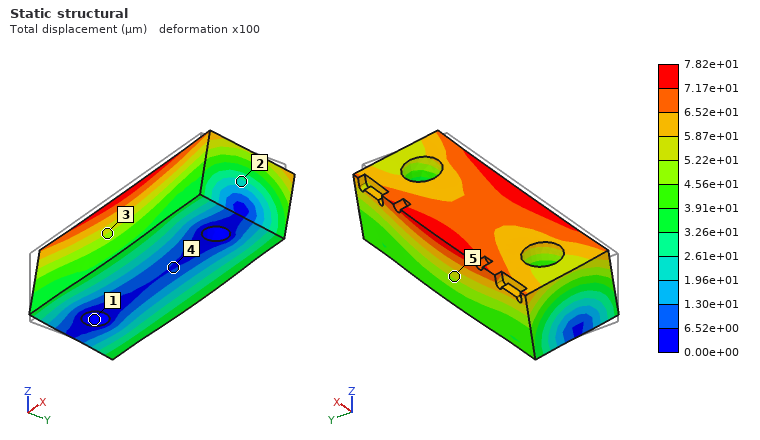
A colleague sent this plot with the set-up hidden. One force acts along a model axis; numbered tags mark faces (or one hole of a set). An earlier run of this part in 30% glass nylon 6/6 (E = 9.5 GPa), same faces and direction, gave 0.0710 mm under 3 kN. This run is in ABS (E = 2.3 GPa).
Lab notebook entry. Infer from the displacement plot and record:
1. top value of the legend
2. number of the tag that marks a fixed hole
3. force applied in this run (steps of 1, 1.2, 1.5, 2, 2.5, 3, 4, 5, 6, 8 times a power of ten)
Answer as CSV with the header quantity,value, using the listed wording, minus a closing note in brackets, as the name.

quantity,value
top value of the legend,7.82e+01 µm
number of the tag that marks a fixed hole,1
force applied in this run,800 N
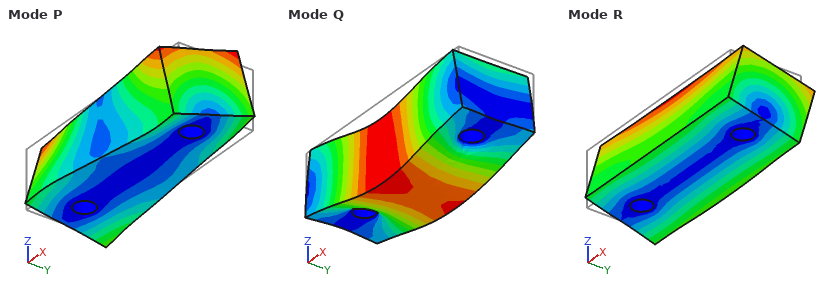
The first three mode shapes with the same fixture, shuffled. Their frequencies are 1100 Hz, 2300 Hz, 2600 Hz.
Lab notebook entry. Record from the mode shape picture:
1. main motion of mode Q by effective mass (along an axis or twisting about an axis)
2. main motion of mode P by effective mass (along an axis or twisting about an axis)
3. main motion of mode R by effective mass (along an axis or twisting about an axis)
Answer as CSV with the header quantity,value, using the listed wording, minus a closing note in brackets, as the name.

quantity,value
main motion of mode Q by effective mass,along Z
main motion of mode P by effective mass,twisting about Z
main motion of mode R by effective mass,along Y
